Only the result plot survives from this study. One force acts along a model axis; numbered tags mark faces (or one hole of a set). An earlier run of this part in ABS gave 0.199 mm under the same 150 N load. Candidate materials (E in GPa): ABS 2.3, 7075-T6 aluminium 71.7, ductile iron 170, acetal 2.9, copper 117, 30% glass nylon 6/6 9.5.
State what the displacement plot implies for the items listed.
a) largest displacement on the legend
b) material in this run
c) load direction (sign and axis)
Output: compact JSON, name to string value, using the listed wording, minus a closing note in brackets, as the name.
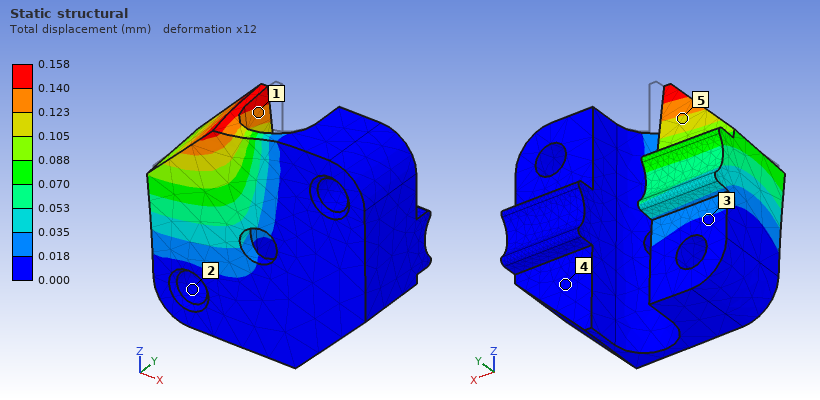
{"largest displacement on the legend": "0.158 mm", "material in this run": "acetal", "load direction": "-Y"}
